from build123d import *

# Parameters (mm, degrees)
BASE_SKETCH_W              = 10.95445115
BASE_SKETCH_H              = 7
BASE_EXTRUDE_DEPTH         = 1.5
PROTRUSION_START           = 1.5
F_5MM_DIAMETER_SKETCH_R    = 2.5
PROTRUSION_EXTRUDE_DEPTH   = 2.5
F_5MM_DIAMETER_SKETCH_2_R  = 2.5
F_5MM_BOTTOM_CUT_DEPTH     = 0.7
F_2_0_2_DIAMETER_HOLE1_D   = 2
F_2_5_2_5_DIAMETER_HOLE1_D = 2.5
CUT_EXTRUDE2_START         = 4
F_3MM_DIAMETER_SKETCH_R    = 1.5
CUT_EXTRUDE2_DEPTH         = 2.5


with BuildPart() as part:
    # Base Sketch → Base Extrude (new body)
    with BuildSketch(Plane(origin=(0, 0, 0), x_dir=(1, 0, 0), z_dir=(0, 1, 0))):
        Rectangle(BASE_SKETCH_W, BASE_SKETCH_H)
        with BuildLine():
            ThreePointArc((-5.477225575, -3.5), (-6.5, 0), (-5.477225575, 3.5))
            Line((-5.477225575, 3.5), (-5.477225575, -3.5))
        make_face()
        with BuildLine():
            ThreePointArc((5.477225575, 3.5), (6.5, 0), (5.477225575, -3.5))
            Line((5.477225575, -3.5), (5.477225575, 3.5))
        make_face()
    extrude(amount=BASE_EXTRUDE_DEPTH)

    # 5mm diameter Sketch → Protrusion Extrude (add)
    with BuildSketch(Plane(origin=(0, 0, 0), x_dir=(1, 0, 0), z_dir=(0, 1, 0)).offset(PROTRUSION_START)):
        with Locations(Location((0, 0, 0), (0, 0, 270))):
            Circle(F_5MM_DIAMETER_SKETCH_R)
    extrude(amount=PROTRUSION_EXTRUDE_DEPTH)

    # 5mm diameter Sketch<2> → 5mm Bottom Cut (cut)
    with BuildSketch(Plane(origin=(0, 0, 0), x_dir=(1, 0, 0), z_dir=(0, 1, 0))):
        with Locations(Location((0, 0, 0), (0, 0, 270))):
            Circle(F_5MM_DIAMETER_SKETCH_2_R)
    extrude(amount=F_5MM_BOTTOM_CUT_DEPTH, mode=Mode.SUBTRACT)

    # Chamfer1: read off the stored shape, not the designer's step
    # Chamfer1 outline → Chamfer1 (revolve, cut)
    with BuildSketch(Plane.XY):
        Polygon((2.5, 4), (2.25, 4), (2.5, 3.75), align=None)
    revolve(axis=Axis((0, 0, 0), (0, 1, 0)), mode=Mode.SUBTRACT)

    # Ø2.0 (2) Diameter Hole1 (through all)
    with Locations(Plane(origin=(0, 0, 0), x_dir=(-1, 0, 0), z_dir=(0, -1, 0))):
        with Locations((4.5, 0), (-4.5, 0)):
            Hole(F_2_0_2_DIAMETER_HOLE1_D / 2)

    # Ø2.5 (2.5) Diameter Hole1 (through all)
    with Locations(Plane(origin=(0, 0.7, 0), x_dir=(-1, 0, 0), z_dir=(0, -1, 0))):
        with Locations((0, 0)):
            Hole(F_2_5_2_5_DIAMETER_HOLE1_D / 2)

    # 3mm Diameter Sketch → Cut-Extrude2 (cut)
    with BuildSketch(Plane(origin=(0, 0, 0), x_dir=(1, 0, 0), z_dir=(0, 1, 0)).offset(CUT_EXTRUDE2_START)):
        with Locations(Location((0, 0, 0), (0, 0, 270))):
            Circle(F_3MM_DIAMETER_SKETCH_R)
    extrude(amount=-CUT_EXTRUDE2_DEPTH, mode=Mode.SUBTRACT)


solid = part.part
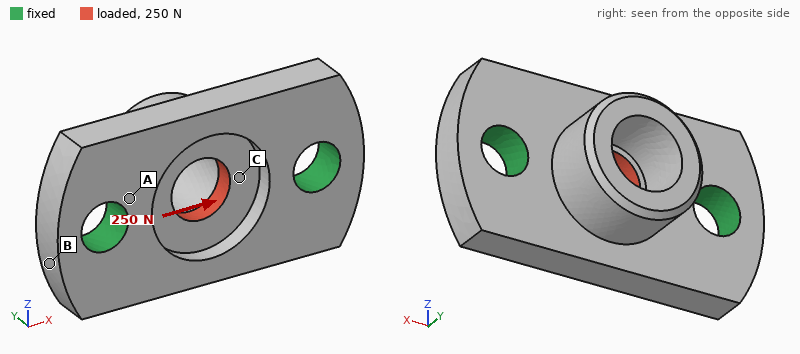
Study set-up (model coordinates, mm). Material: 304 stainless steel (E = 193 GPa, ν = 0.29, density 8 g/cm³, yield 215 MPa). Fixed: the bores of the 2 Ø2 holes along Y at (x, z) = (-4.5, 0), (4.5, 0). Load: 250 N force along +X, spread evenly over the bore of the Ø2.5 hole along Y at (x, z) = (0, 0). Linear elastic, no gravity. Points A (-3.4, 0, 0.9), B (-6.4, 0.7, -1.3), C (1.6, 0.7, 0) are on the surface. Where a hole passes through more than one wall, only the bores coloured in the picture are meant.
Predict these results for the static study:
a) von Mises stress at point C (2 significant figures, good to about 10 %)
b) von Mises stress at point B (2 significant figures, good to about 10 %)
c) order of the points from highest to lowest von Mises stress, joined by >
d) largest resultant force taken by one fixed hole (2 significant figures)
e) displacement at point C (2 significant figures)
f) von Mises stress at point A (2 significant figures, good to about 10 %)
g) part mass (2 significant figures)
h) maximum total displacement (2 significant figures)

47 MPa
7.4 MPa
C > A > B
130 N
0.39 µm
13 MPa
1.1 g
0.61 µm
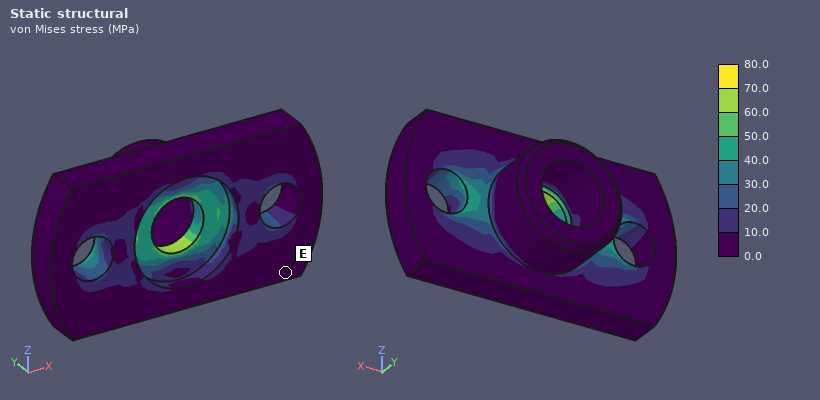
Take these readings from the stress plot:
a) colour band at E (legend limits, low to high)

0.0 to 10.0 MPa
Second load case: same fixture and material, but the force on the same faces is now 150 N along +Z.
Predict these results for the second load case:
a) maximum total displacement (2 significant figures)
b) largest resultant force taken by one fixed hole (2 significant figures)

0.68 µm
75 N
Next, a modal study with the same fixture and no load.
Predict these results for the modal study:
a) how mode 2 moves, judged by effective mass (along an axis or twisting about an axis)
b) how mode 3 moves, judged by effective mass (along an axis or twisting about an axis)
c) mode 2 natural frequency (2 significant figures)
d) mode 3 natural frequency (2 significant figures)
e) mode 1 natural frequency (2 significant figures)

along Y
along X
83 kHz
120 kHz
58 kHz
